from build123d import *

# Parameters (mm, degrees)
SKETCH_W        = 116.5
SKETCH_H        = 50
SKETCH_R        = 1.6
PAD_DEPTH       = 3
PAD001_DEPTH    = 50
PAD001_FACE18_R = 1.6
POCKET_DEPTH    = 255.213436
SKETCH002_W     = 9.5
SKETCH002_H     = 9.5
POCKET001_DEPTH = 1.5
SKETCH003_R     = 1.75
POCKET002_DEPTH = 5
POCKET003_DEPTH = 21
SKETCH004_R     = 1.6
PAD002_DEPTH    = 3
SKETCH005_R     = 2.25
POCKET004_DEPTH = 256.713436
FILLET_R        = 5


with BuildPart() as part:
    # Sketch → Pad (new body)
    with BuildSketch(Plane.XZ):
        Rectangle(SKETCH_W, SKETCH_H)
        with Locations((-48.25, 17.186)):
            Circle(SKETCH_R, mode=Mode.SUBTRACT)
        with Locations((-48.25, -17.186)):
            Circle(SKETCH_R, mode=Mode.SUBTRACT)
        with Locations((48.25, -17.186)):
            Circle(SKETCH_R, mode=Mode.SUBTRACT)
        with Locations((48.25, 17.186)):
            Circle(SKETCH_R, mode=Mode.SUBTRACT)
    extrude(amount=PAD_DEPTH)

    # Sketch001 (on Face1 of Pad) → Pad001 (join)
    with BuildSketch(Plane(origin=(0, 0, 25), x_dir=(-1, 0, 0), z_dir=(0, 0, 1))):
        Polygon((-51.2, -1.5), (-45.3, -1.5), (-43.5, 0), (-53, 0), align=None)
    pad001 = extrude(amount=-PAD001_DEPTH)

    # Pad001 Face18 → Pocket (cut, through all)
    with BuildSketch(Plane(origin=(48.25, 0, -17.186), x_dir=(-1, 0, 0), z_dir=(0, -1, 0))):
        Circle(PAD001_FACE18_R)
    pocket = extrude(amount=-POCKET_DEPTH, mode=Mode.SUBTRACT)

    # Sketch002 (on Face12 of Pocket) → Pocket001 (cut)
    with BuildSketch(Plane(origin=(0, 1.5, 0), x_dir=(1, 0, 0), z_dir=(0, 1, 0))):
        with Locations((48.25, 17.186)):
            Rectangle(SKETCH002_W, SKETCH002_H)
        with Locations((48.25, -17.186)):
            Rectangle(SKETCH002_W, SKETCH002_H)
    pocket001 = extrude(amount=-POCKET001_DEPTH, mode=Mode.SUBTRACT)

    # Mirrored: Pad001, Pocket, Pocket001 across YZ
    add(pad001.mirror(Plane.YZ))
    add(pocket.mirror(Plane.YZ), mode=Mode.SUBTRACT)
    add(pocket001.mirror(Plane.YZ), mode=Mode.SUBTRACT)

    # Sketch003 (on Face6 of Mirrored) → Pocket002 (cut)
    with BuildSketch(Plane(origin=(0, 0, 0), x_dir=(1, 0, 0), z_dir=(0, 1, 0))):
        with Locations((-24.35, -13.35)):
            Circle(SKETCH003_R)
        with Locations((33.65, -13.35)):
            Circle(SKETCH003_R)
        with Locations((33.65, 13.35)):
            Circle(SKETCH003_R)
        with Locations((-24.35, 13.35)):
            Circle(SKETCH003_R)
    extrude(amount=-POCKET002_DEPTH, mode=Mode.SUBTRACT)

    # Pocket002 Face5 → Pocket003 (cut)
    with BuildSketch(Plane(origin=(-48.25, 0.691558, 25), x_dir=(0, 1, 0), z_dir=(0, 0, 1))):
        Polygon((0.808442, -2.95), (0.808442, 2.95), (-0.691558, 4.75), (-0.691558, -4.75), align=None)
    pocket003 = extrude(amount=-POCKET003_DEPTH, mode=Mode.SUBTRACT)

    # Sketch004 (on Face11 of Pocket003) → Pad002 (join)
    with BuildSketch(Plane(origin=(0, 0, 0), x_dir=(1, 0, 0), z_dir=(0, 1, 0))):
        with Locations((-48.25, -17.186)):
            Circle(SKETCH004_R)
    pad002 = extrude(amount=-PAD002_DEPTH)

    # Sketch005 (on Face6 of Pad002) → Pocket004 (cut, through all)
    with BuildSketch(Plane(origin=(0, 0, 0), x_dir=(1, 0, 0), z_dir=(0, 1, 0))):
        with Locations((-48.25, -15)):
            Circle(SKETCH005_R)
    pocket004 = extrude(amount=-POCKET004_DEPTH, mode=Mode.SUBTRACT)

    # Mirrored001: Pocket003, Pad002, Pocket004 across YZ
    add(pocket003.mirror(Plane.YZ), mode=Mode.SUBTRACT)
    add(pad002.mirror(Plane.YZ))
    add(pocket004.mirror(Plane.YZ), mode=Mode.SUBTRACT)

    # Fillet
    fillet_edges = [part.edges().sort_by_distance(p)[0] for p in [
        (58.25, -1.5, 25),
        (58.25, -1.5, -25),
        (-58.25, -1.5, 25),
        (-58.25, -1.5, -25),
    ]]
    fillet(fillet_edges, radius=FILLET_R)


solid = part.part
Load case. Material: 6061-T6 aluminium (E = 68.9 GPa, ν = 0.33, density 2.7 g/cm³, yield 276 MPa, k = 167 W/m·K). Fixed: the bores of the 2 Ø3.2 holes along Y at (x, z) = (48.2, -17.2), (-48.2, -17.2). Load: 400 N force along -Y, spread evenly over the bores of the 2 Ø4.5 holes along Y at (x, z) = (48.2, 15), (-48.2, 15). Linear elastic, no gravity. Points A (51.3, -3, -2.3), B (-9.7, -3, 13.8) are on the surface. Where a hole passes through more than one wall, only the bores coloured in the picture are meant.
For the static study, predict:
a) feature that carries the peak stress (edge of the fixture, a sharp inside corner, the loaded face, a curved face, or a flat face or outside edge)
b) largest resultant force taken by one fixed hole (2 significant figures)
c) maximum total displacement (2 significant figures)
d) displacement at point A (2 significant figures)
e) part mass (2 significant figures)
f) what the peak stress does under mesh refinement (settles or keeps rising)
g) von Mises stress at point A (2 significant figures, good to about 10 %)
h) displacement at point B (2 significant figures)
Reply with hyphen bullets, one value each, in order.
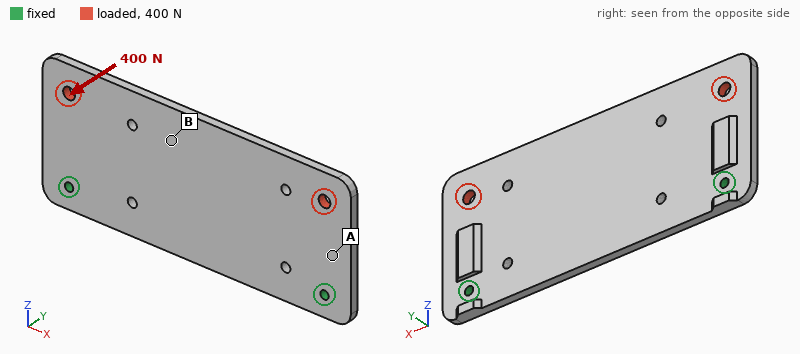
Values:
- edge of the fixture
- 200 N
- 0.64 mm
- 0.15 mm
- 48 g
- keeps rising
- 50 MPa
- 0.40 mm
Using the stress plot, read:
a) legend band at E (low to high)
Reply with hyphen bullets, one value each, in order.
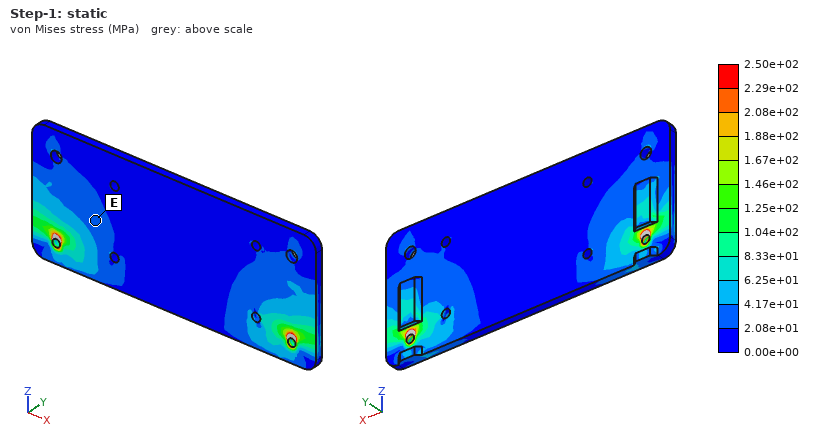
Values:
- 2.08e+01 to 4.17e+01 MPa
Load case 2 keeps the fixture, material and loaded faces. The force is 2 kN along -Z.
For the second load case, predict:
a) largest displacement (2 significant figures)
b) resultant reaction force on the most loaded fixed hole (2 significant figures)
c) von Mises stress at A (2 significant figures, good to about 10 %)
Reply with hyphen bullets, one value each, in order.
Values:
- 17 µm
- 1.0 kN
- 19 MPa
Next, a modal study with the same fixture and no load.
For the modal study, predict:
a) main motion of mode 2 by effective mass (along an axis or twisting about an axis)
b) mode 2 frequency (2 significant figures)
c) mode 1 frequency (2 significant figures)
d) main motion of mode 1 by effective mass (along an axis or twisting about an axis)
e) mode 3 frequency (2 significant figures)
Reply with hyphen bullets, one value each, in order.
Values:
- twisting about Z
- 1700 Hz
- 870 Hz
- along Y
- 1800 Hz
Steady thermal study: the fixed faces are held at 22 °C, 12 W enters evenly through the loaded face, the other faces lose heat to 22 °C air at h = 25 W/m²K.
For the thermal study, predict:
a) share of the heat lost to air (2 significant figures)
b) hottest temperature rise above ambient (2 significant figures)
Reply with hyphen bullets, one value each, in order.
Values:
- 17 %
- 14 K
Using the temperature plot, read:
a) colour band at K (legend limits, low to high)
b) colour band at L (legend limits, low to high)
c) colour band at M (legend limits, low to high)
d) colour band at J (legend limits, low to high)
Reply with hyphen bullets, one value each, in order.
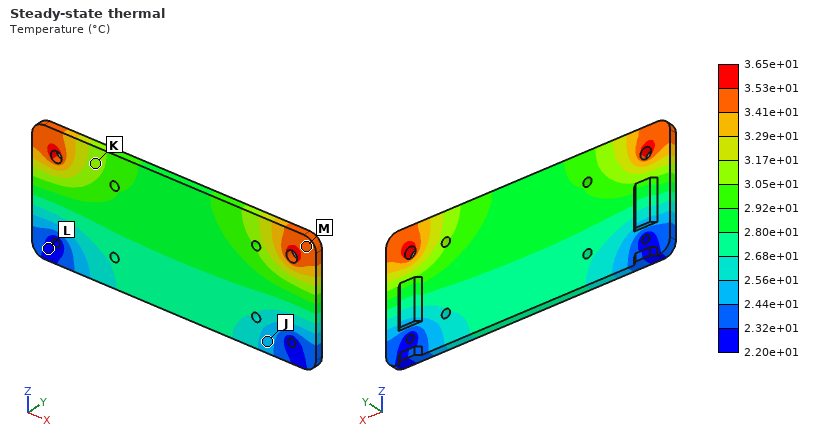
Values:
- 3.05e+01 to 3.17e+01 °C
- 2.20e+01 to 2.32e+01 °C
- 3.41e+01 to 3.53e+01 °C
- 2.44e+01 to 2.56e+01 °C
